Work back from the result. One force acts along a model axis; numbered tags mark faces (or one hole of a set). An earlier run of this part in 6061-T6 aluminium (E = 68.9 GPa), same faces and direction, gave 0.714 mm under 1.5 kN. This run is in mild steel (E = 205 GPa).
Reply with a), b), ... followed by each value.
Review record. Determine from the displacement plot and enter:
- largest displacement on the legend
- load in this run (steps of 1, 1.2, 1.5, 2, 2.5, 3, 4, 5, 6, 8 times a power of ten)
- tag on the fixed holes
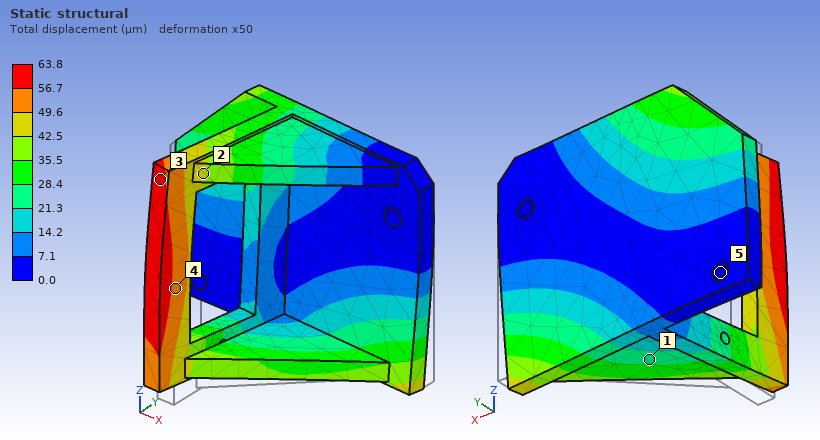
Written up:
a) 63.8 µm
b) 400 N
c) 5
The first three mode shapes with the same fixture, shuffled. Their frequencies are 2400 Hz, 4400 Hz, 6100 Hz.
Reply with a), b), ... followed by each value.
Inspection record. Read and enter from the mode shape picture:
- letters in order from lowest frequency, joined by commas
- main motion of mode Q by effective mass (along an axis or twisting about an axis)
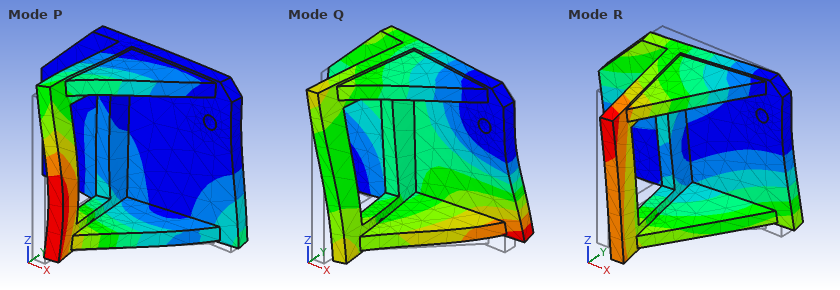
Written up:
a) R, Q, P
b) along Y
